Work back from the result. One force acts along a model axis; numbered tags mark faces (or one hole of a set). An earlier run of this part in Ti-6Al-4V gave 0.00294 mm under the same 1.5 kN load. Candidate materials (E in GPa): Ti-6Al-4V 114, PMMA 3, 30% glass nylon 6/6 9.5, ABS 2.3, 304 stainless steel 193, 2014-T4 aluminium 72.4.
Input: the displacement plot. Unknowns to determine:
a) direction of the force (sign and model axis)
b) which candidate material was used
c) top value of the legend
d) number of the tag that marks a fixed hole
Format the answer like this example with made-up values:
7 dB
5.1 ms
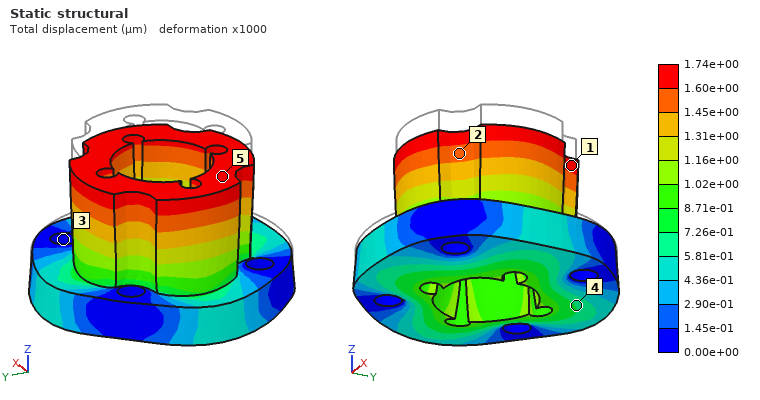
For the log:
-Z
304 stainless steel
1.74e+00 µm
3
